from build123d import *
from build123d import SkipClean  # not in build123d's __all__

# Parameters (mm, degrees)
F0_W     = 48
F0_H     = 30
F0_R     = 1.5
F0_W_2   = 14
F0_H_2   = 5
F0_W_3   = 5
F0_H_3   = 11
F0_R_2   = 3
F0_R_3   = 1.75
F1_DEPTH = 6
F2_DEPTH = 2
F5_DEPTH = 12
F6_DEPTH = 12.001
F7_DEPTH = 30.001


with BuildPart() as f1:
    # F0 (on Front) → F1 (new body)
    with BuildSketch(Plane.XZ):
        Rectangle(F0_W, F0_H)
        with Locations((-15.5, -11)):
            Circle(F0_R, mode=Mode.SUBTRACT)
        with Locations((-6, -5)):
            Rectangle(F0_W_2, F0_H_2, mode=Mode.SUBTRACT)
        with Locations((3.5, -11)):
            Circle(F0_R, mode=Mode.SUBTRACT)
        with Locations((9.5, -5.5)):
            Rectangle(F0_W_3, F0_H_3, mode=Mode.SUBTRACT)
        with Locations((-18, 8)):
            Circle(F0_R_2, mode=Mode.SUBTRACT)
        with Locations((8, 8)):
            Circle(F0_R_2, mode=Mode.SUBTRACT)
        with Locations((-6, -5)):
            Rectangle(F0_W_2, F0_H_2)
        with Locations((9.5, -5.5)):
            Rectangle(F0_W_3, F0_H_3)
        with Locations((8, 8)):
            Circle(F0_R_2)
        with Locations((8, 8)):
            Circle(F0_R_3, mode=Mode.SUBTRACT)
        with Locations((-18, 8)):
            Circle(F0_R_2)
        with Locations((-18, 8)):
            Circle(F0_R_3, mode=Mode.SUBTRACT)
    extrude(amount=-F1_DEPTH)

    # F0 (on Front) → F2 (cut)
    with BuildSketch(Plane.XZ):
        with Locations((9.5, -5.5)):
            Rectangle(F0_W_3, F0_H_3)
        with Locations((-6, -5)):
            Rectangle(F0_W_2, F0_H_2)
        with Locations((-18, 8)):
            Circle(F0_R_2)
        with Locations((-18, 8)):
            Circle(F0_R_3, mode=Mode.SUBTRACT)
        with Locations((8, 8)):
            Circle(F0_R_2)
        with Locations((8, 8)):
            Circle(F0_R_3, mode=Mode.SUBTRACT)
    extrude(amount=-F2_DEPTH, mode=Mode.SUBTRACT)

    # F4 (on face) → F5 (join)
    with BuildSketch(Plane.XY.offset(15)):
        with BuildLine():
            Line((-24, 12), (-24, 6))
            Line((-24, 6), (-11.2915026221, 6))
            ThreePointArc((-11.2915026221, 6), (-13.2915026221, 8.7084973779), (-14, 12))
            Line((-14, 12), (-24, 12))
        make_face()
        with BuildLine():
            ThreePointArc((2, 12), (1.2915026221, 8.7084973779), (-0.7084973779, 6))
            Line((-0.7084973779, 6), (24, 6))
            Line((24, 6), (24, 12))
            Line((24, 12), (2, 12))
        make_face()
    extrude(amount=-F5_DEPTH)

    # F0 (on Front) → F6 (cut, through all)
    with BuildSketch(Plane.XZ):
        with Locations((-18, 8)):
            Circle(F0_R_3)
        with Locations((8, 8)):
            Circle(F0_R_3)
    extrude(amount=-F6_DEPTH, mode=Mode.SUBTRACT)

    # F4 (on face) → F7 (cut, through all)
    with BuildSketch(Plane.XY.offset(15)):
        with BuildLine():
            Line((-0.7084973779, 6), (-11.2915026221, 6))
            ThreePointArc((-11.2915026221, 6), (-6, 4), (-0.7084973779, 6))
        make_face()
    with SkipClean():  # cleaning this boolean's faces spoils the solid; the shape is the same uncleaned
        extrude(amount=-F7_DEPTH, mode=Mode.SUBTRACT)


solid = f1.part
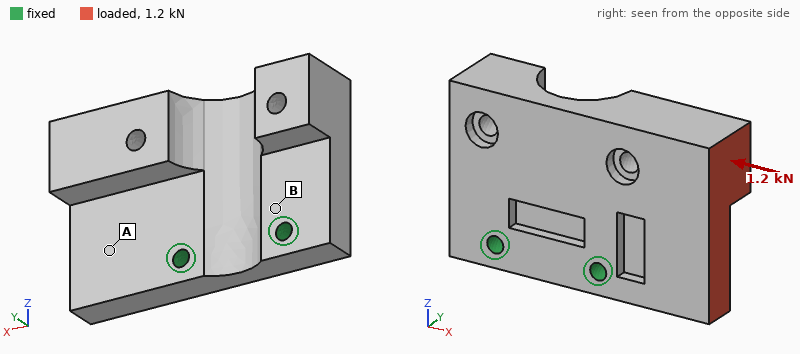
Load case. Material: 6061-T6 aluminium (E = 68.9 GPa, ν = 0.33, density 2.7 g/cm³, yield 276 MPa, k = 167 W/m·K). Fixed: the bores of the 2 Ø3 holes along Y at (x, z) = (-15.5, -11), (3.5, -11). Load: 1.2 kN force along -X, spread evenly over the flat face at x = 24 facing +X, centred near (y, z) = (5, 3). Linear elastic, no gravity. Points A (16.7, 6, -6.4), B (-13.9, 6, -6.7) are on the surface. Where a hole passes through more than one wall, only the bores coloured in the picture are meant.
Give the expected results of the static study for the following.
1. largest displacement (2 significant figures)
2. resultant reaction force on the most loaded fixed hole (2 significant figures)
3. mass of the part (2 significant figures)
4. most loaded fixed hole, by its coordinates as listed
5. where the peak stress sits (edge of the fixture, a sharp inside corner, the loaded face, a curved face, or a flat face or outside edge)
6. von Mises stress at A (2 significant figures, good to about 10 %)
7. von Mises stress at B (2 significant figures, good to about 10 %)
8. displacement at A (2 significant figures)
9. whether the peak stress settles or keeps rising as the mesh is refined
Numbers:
32 µm
1.0 kN
27 g
(3.5, -11)
edge of the fixture
8.0 MPa
15 MPa
11 µm
keeps rising
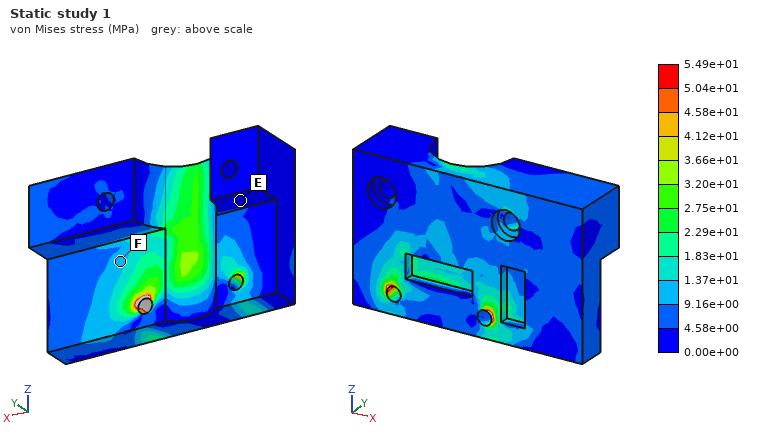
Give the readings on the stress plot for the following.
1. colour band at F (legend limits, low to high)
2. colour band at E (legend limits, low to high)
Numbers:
9.16e+00 to 1.37e+01 MPa
0.00e+00 to 4.58e+00 MPa
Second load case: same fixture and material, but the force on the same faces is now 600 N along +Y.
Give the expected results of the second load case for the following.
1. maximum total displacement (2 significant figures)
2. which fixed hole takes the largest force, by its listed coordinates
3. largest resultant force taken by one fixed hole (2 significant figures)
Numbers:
0.19 mm
(3.5, -11)
880 N
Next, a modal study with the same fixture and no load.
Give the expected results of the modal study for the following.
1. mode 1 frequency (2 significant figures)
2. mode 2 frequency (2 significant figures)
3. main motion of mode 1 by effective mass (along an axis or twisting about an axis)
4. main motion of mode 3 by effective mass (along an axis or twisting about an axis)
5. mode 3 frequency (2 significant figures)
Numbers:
3500 Hz
5800 Hz
along Y
along X
9500 Hz
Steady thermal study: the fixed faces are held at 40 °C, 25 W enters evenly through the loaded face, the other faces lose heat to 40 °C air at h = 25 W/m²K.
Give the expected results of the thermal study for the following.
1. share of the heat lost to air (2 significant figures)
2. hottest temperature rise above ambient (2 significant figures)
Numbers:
4.4 %
24 K
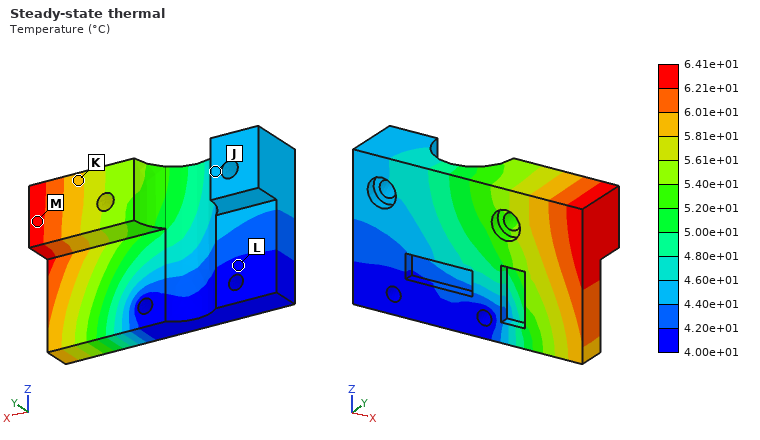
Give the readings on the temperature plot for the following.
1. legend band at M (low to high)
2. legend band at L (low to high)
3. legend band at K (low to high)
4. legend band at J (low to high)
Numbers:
6.21e+01 to 6.41e+01 °C
4.00e+01 to 4.20e+01 °C
5.81e+01 to 6.01e+01 °C
4.40e+01 to 4.60e+01 °C
